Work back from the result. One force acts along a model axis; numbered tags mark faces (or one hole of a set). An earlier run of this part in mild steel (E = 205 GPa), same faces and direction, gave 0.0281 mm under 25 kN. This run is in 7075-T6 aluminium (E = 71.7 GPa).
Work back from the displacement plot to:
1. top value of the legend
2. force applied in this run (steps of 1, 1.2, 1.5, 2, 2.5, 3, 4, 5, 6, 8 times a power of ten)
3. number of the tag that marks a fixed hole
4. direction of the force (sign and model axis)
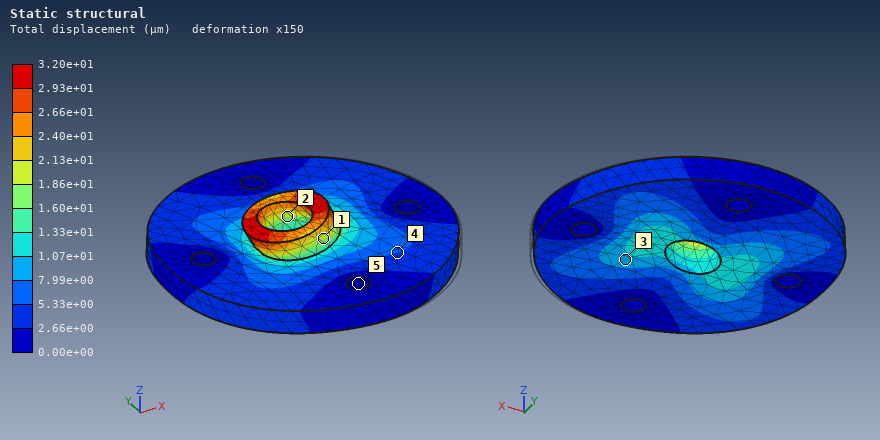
3.20e+01 µm
10 kN
5
-X
